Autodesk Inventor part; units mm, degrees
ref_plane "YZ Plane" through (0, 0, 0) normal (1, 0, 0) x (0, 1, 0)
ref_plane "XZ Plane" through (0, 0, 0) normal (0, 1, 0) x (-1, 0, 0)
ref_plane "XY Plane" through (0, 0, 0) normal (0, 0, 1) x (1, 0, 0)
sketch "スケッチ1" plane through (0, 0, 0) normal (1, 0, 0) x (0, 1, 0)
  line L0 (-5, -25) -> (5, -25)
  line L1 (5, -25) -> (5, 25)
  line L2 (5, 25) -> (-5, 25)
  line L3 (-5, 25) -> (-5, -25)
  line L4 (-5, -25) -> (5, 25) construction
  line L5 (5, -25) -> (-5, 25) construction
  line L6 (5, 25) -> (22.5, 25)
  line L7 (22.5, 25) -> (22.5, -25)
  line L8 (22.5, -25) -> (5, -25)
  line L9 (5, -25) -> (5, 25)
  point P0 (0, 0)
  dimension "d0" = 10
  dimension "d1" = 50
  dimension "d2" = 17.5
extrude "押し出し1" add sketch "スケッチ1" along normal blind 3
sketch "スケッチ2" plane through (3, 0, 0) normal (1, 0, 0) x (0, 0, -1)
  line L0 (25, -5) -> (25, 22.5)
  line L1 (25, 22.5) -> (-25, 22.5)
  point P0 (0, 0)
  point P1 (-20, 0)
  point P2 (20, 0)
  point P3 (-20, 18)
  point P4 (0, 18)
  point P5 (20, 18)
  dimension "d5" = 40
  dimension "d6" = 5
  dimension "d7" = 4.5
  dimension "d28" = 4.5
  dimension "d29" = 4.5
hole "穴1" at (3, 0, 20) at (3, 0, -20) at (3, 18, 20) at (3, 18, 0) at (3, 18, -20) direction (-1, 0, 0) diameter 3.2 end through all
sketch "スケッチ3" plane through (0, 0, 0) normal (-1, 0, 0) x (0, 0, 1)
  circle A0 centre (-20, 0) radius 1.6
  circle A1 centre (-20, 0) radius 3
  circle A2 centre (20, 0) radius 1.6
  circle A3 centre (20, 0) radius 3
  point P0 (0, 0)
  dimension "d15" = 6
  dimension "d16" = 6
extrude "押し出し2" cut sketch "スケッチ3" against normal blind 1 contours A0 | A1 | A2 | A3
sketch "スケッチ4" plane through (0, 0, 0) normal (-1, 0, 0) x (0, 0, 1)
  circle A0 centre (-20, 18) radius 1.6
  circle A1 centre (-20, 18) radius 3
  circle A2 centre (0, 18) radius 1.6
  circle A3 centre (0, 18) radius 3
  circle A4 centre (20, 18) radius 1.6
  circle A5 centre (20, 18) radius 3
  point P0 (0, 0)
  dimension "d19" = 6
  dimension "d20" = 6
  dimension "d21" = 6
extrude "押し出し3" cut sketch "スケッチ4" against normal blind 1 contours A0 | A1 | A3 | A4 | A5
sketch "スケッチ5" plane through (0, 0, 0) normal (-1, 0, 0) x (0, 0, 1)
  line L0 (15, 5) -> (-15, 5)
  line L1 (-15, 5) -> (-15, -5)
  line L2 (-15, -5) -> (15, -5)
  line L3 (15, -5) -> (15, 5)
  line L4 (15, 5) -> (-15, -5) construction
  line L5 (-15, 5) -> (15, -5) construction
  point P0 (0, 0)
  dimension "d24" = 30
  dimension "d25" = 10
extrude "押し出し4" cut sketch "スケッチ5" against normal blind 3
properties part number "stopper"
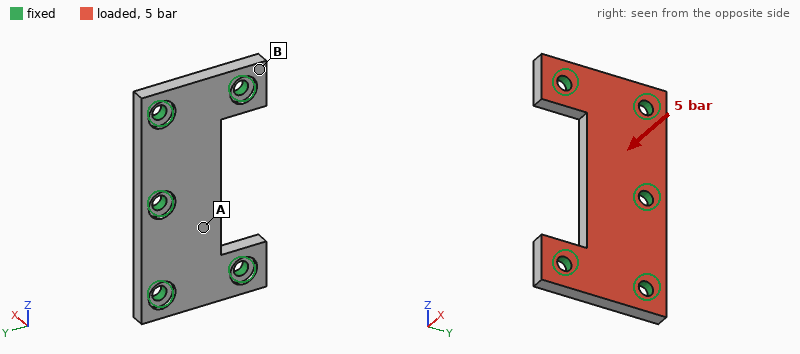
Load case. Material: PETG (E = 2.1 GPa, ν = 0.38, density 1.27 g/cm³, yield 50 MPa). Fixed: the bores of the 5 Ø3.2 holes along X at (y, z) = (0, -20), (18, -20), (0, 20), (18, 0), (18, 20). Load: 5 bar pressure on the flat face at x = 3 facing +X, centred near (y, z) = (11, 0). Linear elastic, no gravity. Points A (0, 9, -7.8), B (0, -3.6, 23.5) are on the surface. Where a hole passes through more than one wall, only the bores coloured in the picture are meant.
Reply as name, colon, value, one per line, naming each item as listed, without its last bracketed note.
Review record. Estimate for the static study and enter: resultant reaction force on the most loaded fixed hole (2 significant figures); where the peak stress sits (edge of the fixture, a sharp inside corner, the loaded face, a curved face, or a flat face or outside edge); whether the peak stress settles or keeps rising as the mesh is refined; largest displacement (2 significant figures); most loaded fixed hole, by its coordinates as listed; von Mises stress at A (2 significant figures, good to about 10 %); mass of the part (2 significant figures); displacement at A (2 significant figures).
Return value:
resultant reaction force on the most loaded fixed hole: 160 N
where the peak stress sits: edge of the fixture
whether the peak stress settles or keeps rising as the mesh is refined: keeps rising
largest displacement: 0.36 mm
most loaded fixed hole, by its coordinates as listed: (18, 0)
von Mises stress at A: 10 MPa
mass of the part: 3.8 g
displacement at A: 0.22 mm
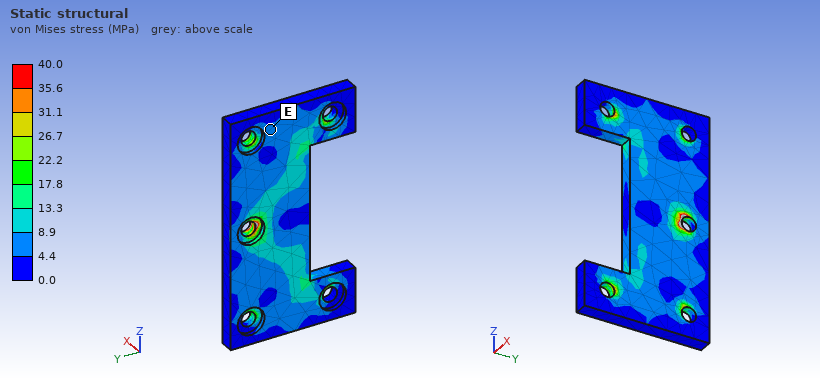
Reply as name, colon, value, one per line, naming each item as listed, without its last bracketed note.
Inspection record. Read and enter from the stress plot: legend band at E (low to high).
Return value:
legend band at E: 4.4 to 8.9 MPa
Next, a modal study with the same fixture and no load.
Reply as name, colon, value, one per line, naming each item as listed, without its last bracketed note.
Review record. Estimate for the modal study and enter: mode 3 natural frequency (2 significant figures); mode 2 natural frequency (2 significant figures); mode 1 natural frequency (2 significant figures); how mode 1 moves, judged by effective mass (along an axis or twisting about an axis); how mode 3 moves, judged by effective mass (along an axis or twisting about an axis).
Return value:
mode 3 natural frequency: 8800 Hz
mode 2 natural frequency: 6300 Hz
mode 1 natural frequency: 4000 Hz
how mode 1 moves, judged by effective mass: along X
how mode 3 moves, judged by effective mass: along X
